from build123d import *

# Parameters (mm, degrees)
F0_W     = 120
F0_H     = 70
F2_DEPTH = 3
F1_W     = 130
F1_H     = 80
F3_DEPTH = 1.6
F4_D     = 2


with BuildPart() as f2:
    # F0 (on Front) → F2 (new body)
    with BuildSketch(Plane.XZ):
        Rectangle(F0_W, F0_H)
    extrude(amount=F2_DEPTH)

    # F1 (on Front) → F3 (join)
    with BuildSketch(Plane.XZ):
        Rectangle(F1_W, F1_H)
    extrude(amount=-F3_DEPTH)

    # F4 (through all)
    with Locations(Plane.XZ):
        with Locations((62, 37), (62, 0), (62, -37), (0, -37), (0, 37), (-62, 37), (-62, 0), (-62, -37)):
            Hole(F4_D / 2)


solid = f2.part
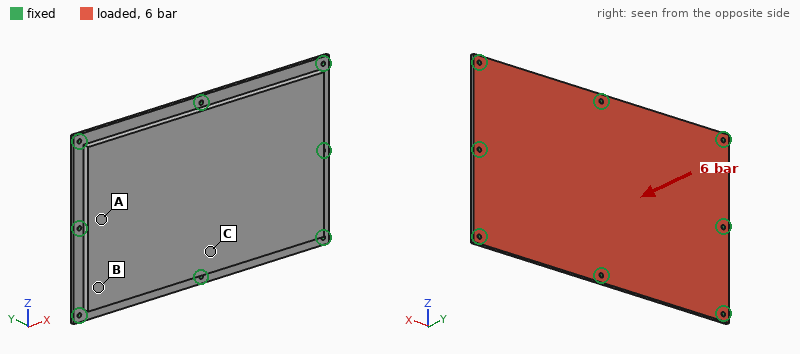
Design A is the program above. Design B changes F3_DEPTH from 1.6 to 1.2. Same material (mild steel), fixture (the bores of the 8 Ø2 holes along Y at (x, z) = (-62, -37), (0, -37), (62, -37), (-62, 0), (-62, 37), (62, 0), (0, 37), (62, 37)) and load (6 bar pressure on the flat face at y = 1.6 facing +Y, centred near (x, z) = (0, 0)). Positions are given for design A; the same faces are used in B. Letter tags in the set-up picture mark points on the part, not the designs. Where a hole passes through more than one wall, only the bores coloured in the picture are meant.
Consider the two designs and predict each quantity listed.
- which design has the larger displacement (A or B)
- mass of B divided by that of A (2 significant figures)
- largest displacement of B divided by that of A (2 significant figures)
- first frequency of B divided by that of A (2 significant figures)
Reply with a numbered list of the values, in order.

1. B
2. 0.90
3. 1.3
4. 0.91
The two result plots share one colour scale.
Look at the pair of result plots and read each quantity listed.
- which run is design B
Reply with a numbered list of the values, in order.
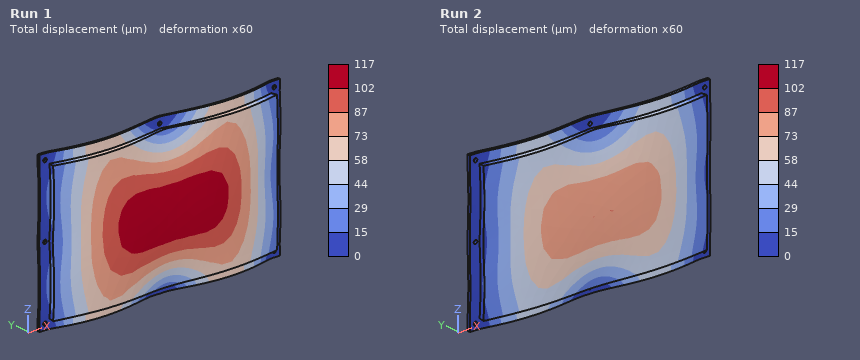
1. Run 1
